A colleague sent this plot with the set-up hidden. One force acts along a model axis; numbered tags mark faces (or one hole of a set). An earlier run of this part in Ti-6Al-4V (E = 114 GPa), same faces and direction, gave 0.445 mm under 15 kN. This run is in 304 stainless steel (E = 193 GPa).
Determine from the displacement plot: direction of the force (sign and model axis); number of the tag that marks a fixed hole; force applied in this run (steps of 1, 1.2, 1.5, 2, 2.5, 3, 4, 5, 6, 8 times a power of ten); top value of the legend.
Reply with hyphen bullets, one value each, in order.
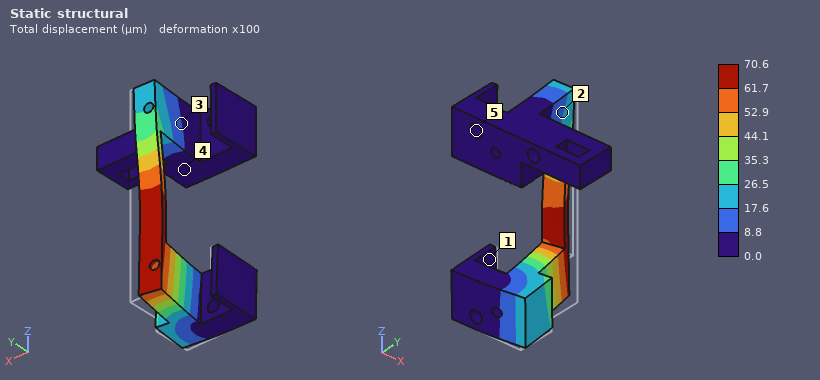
- -X
- 5
- 4 kN
- 70.6 µm
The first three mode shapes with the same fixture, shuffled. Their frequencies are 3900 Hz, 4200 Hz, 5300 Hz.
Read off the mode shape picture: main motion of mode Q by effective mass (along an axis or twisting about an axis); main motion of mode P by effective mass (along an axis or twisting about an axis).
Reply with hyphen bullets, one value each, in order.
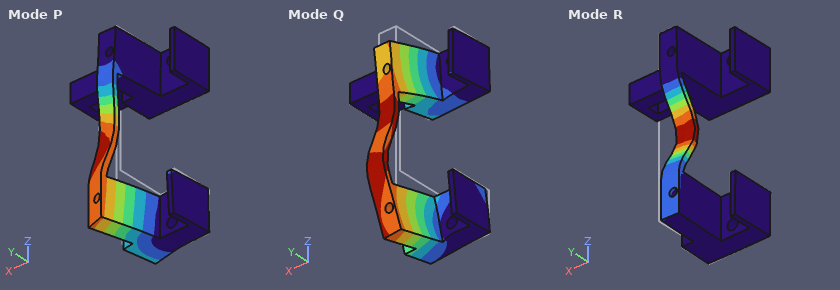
- along Z
- along X
